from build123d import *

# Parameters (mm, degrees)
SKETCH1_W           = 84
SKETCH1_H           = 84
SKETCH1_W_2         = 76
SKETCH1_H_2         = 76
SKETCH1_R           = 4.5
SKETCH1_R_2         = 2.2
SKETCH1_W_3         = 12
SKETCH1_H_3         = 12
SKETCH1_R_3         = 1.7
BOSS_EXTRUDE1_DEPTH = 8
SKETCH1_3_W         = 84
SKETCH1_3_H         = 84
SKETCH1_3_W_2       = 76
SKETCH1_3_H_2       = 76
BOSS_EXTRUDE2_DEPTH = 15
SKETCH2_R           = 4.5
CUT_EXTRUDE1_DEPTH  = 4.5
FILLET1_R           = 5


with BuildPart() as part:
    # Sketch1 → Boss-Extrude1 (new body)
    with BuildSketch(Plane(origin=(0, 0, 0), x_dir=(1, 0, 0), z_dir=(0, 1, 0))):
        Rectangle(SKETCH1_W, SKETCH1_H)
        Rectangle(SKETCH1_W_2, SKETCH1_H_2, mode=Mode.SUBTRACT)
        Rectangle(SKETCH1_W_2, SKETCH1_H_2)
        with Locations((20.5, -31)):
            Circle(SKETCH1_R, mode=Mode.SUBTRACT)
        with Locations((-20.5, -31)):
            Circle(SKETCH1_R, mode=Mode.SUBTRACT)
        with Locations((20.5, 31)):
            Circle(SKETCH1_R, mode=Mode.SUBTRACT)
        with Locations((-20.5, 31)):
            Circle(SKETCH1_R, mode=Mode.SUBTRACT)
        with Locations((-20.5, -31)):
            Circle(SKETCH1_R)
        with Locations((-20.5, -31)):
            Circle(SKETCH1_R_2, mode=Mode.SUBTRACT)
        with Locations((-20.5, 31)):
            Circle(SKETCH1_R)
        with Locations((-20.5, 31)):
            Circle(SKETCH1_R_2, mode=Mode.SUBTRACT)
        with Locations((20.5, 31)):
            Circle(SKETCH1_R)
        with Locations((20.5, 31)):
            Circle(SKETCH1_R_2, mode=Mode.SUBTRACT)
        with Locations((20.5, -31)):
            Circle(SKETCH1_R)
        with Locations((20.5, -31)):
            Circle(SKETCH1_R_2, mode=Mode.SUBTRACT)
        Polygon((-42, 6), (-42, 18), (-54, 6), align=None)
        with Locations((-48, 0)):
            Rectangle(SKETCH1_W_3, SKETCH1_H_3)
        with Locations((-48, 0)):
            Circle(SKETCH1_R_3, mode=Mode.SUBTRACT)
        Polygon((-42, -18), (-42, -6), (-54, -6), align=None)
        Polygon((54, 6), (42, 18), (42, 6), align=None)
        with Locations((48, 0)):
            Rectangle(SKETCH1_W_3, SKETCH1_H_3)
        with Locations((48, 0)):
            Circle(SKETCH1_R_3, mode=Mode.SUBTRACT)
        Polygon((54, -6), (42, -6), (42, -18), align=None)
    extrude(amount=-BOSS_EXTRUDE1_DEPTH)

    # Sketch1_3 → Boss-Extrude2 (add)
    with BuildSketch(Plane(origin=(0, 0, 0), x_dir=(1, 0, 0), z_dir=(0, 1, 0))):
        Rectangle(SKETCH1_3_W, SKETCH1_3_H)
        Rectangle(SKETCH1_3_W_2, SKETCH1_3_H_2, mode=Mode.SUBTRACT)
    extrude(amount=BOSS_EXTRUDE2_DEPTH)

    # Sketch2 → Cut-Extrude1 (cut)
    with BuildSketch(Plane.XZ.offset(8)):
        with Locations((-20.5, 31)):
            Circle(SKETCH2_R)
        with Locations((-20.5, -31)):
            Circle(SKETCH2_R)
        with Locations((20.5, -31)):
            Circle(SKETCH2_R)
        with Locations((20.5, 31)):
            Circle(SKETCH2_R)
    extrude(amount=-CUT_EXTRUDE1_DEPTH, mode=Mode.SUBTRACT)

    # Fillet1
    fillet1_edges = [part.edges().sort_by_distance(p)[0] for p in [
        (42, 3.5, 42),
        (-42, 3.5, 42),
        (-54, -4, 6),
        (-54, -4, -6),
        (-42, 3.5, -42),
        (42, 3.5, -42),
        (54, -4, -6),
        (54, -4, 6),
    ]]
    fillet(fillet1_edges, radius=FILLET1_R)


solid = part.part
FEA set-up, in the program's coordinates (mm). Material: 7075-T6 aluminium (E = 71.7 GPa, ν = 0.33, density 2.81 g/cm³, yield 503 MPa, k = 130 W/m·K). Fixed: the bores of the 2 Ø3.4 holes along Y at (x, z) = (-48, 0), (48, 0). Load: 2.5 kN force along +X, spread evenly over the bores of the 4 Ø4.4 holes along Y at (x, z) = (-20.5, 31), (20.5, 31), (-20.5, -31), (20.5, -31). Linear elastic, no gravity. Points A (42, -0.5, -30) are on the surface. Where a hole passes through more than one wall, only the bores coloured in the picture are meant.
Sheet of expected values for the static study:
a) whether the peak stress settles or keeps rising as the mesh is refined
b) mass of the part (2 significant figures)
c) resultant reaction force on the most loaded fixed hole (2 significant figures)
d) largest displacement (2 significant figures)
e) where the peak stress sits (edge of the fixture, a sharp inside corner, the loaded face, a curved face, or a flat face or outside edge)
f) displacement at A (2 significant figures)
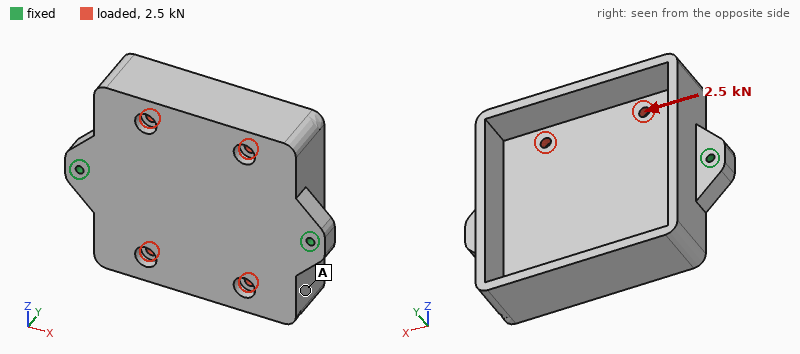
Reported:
keeps rising
220 g
1.3 kN
5.2 µm
edge of the fixture
4.0 µm
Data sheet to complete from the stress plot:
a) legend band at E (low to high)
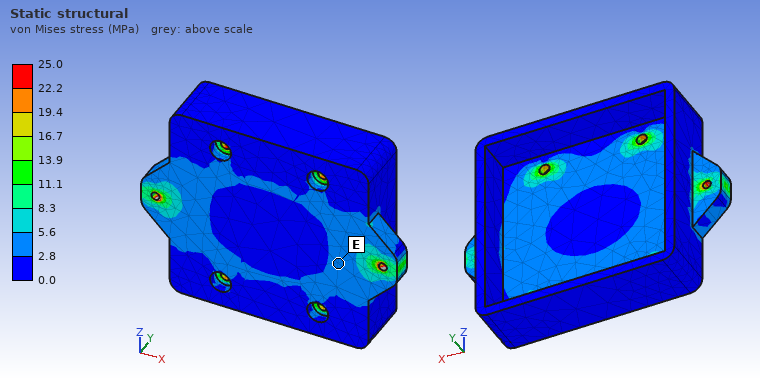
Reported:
2.8 to 5.6 MPa
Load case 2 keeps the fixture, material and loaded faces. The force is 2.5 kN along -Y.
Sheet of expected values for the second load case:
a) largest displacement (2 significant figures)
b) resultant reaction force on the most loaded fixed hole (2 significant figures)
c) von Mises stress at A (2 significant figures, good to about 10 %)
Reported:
51 µm
1.3 kN
14 MPa
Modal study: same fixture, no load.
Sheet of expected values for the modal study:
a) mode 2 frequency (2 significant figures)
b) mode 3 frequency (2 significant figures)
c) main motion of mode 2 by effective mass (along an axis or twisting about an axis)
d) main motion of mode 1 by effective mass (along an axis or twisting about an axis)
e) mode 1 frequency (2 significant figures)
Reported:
3100 Hz
3700 Hz
along Y
twisting about X
1600 Hz
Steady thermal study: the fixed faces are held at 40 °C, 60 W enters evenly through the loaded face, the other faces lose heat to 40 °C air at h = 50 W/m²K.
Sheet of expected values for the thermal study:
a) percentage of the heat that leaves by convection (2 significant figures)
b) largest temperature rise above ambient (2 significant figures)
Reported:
34 %
25 K
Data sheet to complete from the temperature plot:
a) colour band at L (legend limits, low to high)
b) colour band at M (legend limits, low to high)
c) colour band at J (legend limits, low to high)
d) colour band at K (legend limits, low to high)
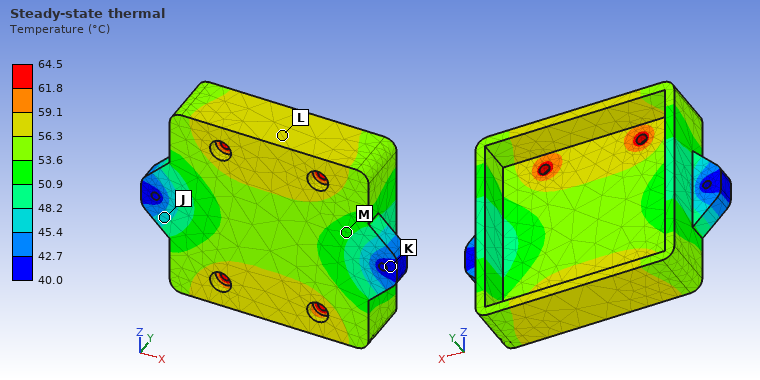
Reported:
56.3 to 59.1 °C
50.9 to 53.6 °C
45.4 to 48.2 °C
40.0 to 42.7 °C
